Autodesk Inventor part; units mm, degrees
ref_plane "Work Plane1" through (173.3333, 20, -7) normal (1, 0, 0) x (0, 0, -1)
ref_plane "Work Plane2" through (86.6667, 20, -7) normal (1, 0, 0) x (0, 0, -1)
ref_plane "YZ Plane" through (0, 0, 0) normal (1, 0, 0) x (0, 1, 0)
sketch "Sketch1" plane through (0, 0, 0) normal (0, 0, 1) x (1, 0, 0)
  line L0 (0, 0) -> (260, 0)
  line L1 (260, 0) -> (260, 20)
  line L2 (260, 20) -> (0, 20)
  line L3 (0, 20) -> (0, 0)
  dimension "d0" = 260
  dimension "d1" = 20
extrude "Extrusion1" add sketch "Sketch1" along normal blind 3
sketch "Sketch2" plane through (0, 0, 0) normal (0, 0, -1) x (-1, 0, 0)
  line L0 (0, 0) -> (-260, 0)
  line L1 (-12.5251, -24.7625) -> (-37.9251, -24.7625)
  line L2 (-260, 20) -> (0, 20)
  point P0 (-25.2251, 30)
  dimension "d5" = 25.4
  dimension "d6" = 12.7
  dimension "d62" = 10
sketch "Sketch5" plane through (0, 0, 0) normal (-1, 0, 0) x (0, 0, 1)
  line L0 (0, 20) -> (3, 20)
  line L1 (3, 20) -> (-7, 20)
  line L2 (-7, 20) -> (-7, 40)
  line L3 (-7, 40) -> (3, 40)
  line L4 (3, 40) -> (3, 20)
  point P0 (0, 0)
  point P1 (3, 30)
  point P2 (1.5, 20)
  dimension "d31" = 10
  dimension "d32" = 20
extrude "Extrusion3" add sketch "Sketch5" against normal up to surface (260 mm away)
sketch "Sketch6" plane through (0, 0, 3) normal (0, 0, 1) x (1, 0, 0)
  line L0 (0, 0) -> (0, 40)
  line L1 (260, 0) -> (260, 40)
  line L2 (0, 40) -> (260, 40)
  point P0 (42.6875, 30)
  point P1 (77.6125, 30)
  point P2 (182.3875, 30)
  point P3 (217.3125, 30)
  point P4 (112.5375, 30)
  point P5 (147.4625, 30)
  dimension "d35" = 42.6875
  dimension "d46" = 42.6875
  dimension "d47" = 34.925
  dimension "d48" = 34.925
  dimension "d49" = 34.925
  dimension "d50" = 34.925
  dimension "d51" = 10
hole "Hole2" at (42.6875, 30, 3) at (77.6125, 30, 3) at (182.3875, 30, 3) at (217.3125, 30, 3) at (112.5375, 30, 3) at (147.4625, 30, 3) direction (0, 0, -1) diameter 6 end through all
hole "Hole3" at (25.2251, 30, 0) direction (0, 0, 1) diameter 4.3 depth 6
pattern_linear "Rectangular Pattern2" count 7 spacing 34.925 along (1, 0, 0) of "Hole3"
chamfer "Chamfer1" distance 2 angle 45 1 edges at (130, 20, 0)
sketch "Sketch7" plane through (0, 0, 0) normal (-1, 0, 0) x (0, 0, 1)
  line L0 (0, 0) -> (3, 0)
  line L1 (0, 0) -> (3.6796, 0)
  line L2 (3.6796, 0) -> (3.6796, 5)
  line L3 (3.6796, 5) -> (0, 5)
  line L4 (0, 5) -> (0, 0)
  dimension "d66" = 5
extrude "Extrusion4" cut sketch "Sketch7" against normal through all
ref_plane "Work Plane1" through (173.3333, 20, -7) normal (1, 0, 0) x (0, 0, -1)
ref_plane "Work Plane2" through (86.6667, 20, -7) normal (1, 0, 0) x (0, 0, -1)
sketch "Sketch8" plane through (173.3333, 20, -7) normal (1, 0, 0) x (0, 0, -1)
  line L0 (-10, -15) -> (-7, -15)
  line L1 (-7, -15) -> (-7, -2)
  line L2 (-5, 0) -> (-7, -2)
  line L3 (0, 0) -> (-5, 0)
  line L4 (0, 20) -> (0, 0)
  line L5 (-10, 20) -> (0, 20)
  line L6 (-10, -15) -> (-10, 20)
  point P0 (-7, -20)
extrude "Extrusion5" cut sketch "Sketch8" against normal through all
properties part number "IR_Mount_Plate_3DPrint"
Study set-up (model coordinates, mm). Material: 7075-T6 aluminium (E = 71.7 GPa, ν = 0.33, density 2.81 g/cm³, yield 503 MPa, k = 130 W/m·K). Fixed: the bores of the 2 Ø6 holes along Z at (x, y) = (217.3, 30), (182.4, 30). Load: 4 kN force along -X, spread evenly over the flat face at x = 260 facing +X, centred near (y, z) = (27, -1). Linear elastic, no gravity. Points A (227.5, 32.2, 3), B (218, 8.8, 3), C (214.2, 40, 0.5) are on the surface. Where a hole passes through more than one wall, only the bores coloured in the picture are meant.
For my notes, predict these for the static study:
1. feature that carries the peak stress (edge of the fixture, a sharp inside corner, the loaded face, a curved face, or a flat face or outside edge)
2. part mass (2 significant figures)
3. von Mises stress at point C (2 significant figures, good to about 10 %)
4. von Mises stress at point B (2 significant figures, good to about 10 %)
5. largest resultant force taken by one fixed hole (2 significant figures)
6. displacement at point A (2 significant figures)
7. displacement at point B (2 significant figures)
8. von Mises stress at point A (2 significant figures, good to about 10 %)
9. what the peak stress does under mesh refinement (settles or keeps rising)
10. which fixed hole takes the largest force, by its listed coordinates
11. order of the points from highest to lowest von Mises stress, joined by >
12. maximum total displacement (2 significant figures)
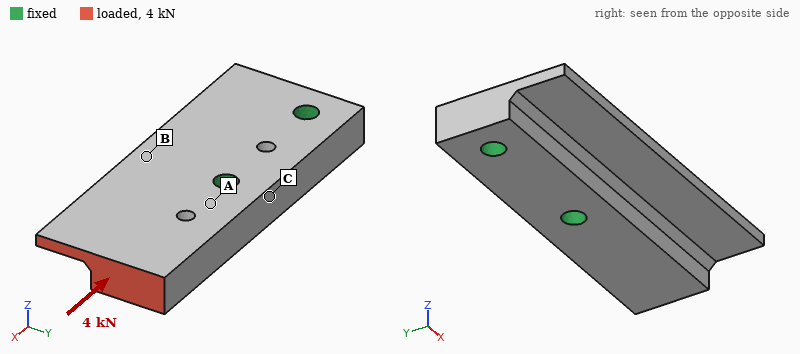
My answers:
edge of the fixture
58 g
5.7 MPa
13 MPa
3.5 kN
2.7 µm
5.4 µm
21 MPa
keeps rising
(217.3, 30)
A > B > C
17 µm
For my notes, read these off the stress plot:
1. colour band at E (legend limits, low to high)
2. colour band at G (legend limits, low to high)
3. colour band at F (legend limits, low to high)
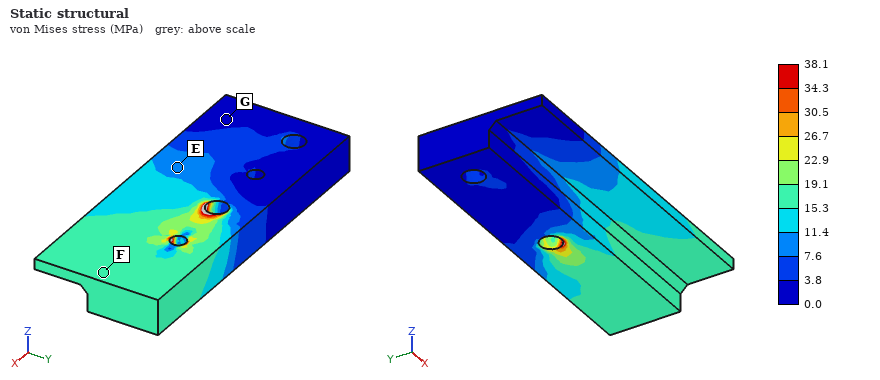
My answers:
7.6 to 11.4 MPa
0.0 to 3.8 MPa
15.3 to 19.1 MPa
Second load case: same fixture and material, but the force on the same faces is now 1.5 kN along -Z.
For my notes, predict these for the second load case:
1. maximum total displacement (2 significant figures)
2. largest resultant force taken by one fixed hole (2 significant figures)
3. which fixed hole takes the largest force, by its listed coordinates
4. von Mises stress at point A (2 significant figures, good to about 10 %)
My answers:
0.39 mm
1.9 kN
(217.3, 30)
130 MPa
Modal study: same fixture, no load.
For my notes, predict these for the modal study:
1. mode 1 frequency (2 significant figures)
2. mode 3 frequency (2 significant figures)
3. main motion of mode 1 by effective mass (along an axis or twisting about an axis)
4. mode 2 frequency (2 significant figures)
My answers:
4000 Hz
7800 Hz
along Z
7500 Hz
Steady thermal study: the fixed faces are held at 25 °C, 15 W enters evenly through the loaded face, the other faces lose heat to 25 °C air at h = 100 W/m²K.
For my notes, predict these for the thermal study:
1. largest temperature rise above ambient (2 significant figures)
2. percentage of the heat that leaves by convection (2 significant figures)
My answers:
18 K
23 %
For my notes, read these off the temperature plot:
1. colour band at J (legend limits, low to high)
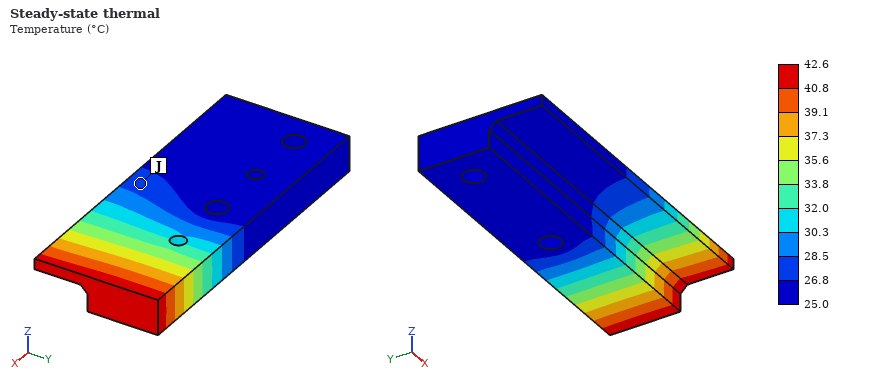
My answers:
26.8 to 28.5 °C
